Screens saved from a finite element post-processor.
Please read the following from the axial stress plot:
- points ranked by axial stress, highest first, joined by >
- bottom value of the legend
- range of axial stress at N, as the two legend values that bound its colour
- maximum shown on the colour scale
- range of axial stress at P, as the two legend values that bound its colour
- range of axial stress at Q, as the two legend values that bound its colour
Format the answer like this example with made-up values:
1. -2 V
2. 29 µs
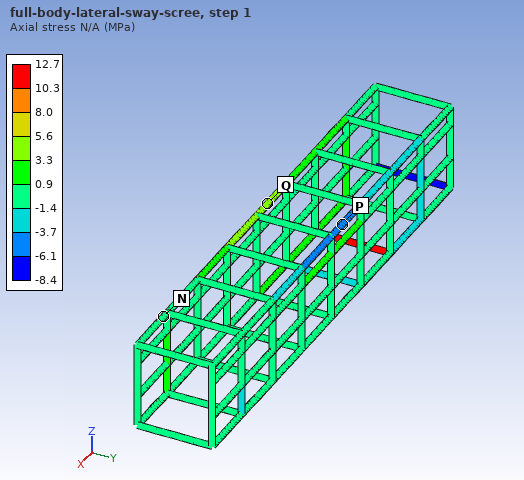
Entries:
1. Q > N > P
2. -8.4 MPa
3. -1.4 to 0.9 MPa
4. 12.7 MPa
5. -6.1 to -3.7 MPa
6. 3.3 to 5.6 MPa
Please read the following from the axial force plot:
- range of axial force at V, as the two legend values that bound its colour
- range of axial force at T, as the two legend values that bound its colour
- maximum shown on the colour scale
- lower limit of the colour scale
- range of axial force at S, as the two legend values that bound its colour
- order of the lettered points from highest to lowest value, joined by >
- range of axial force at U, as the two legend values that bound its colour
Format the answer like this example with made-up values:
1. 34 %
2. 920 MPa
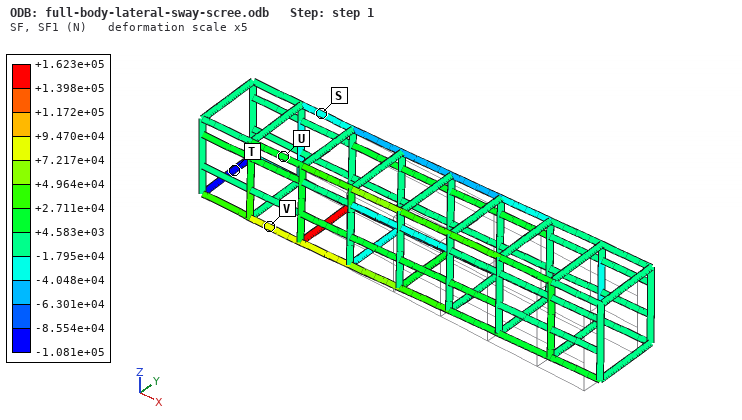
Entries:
1. +7.217e+04 to +9.470e+04 N
2. -1.081e+05 to -8.554e+04 N
3. +1.623e+05 N
4. -1.081e+05 N
5. -4.048e+04 to -1.795e+04 N
6. V > U > S > T
7. +4.583e+03 to +2.711e+04 N
